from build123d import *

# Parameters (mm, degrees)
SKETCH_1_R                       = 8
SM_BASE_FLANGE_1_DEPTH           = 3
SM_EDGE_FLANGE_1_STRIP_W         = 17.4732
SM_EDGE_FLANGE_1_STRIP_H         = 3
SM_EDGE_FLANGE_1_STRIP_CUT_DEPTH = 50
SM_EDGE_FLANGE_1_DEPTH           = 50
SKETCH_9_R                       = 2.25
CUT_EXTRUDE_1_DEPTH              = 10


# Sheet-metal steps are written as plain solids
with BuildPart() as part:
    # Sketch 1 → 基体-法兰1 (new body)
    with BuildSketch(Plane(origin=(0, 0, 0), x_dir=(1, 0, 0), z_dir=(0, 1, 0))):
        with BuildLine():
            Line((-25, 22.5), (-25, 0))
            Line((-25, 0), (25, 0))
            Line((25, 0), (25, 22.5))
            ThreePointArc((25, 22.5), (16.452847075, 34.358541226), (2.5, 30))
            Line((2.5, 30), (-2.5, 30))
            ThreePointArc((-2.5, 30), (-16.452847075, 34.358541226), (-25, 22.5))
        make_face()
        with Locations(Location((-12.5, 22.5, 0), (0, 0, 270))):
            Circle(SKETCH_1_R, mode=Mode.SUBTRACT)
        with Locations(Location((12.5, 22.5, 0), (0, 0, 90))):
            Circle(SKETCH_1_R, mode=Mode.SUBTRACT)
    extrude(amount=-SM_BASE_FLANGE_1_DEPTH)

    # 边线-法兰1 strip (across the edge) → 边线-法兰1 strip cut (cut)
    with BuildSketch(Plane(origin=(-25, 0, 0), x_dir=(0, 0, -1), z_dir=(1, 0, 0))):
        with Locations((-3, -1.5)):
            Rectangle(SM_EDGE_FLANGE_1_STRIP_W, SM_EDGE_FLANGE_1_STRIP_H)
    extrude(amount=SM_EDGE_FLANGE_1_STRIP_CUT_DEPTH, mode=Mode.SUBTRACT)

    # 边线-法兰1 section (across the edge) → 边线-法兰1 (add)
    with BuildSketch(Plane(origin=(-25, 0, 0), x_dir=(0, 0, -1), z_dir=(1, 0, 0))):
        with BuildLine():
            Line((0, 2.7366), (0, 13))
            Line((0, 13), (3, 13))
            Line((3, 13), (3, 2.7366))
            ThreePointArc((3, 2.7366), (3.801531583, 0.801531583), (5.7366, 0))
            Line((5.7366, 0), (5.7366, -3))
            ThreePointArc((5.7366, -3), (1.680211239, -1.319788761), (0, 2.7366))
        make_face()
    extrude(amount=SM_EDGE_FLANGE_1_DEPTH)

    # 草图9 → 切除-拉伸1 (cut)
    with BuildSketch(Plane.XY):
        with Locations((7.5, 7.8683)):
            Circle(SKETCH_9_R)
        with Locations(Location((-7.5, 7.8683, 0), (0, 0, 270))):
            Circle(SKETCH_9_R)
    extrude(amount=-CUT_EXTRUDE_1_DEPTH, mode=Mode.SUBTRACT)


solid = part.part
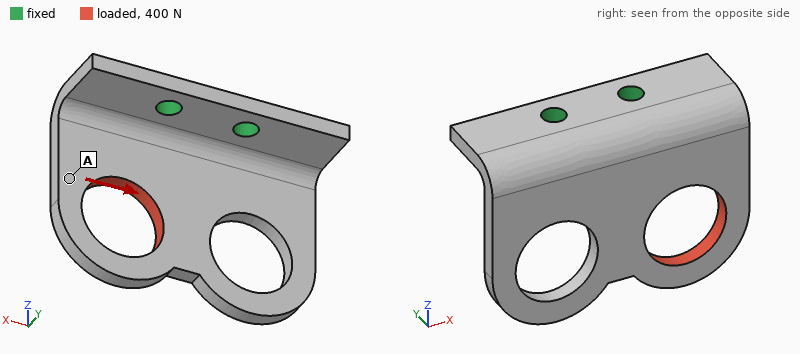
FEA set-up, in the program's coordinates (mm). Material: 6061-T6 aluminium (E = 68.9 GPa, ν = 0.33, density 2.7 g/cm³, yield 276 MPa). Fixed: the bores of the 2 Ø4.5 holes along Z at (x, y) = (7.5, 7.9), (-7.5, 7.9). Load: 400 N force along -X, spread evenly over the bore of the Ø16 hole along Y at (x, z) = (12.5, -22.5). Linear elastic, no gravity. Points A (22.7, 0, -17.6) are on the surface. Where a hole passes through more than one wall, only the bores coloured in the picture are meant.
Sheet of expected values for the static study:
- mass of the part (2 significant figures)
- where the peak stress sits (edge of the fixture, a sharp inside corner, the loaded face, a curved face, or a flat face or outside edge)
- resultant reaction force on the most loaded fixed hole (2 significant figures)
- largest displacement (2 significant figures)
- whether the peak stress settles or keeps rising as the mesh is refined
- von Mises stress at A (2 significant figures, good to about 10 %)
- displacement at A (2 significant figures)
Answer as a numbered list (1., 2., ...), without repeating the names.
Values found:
1. 14 g
2. edge of the fixture
3. 500 N
4. 0.11 mm
5. keeps rising
6. 19 MPa
7. 0.077 mm
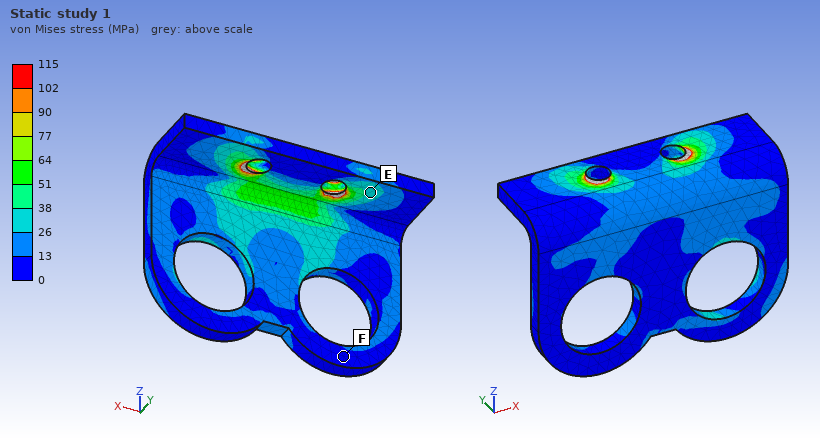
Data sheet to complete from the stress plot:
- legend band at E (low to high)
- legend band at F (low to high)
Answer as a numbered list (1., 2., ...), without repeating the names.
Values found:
1. 26 to 38 MPa
2. 0 to 13 MPa
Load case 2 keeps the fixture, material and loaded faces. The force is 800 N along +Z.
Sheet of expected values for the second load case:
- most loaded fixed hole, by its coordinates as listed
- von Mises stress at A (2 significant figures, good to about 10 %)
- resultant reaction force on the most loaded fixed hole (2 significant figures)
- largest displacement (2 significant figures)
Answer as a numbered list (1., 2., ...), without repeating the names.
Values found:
1. (7.5, 7.9)
2. 29 MPa
3. 890 N
4. 0.26 mm
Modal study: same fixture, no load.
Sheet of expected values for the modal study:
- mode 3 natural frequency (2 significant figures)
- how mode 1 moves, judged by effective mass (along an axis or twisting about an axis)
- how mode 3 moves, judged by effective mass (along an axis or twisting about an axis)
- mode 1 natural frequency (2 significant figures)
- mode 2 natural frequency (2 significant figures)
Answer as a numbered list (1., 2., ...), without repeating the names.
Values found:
1. 5200 Hz
2. along Y
3. along X
4. 2100 Hz
5. 3400 Hz
